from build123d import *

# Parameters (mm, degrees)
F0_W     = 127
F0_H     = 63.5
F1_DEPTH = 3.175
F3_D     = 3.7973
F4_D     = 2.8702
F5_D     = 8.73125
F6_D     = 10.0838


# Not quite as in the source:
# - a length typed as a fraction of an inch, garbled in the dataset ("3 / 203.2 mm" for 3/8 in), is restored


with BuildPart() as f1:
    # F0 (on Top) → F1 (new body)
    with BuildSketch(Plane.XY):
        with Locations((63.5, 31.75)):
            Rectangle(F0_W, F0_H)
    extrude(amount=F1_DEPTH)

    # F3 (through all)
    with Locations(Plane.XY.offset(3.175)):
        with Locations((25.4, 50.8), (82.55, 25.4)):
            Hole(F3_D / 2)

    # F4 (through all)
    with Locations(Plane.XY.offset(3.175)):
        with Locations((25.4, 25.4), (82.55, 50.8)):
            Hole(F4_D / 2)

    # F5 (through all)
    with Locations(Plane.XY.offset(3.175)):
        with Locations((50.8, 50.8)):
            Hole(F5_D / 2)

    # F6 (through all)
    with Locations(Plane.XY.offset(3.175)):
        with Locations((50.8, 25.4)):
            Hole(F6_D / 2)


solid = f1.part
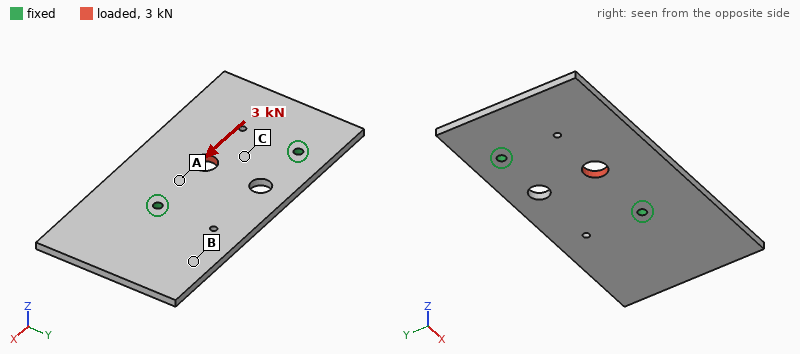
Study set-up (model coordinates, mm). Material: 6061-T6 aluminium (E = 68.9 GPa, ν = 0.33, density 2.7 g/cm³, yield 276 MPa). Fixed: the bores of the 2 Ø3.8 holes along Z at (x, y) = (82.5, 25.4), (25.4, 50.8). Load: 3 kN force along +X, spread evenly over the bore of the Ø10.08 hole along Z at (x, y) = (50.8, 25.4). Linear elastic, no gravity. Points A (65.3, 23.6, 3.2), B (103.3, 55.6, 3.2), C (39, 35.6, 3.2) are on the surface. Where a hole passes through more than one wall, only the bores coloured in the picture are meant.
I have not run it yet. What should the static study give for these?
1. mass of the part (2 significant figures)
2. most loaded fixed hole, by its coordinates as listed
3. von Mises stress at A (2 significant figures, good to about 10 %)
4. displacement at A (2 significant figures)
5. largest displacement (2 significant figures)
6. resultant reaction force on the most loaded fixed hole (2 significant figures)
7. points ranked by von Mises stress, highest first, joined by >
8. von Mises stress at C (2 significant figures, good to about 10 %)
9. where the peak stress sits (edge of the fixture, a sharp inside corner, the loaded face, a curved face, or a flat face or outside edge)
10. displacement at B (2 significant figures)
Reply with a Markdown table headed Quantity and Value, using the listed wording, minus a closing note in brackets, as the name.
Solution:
| Quantity | Value |
|---|---|
| mass of the part | 68 g |
| most loaded fixed hole, by its coordinates as listed | (82.5, 25.4) |
| von Mises stress at A | 29 MPa |
| displacement at A | 8.1 µm |
| largest displacement | 16 µm |
| resultant reaction force on the most loaded fixed hole | 2.0 kN |
| points ranked by von Mises stress, highest first, joined by > | A > C > B |
| von Mises stress at C | 16 MPa |
| where the peak stress sits | edge of the fixture |
| displacement at B | 4.0 µm |
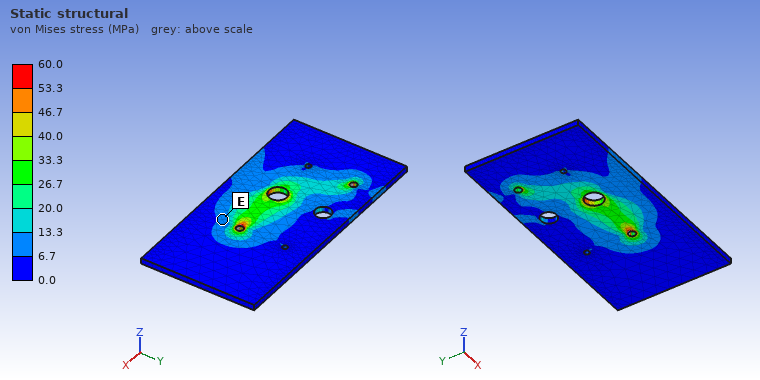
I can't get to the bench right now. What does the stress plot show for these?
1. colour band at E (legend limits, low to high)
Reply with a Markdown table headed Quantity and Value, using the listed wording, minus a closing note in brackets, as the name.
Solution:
| Quantity | Value |
|---|---|
| colour band at E | 6.7 to 13.3 MPa |
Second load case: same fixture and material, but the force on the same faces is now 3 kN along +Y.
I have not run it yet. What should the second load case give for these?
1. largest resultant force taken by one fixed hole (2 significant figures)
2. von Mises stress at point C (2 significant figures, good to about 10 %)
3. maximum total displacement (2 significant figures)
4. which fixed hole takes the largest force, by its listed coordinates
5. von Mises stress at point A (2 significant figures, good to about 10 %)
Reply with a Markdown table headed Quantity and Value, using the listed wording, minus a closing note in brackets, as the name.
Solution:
| Quantity | Value |
|---|---|
| largest resultant force taken by one fixed hole | 1.7 kN |
| von Mises stress at point C | 24 MPa |
| maximum total displacement | 18 µm |
| which fixed hole takes the largest force, by its listed coordinates | (25.4, 50.8) |
| von Mises stress at point A | 13 MPa |
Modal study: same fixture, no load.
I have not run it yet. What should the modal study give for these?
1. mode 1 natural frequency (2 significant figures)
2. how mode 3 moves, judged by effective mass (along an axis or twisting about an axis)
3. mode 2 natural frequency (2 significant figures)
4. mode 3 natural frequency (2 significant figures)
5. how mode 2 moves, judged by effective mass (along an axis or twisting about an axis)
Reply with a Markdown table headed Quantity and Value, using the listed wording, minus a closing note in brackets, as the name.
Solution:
| Quantity | Value |
|---|---|
| mode 1 natural frequency | 980 Hz |
| how mode 3 moves, judged by effective mass | twisting about X |
| mode 2 natural frequency | 1200 Hz |
| mode 3 natural frequency | 1500 Hz |
| how mode 2 moves, judged by effective mass | along Z |
